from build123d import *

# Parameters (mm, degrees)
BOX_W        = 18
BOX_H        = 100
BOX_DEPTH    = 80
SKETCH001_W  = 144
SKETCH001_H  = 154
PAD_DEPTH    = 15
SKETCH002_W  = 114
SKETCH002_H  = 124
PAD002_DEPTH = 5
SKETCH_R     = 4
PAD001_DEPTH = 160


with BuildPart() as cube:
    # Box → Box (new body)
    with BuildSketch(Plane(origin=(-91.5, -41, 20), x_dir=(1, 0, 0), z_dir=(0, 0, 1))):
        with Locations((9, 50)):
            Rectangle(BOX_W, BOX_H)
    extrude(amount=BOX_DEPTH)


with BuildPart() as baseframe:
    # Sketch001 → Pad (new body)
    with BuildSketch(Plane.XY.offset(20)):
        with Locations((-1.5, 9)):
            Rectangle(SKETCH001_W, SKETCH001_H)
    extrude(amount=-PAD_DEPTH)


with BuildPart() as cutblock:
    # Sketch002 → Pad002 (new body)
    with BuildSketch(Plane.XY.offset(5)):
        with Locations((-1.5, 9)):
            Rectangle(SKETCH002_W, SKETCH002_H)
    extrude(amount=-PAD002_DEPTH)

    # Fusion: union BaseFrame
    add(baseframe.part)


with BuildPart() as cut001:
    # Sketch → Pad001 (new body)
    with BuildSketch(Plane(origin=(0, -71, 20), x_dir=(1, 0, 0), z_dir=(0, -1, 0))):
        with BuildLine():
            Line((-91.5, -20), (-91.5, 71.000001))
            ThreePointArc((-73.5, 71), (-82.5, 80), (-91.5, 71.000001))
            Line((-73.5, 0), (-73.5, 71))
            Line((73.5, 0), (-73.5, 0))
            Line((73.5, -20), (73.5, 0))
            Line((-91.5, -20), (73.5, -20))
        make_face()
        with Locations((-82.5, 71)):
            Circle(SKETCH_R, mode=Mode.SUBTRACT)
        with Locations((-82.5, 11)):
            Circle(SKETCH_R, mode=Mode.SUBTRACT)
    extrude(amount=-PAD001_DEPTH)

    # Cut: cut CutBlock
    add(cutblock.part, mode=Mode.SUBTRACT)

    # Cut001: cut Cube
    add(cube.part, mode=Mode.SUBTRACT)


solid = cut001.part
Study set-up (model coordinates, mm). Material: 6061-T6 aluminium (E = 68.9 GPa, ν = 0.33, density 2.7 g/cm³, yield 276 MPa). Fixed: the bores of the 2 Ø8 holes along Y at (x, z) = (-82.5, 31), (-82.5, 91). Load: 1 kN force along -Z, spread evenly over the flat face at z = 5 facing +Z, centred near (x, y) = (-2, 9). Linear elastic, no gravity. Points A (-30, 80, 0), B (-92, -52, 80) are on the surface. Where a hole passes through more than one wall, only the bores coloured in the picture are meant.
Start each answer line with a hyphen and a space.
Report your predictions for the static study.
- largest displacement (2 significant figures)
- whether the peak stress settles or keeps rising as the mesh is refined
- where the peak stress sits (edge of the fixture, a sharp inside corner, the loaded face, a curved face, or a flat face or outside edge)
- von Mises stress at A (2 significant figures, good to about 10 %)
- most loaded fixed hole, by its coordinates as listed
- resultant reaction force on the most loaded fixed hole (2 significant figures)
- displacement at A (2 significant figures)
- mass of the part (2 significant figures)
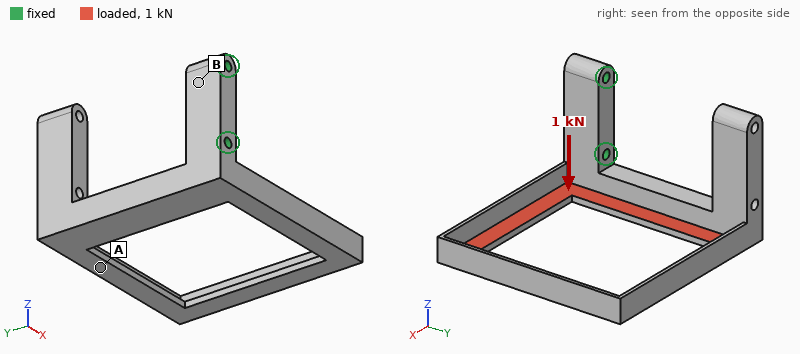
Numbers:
- 2.9 mm
- keeps rising
- a sharp inside corner
- 25 MPa
- (-82.5, 31)
- 1.0 kN
- 1.1 mm
- 550 g
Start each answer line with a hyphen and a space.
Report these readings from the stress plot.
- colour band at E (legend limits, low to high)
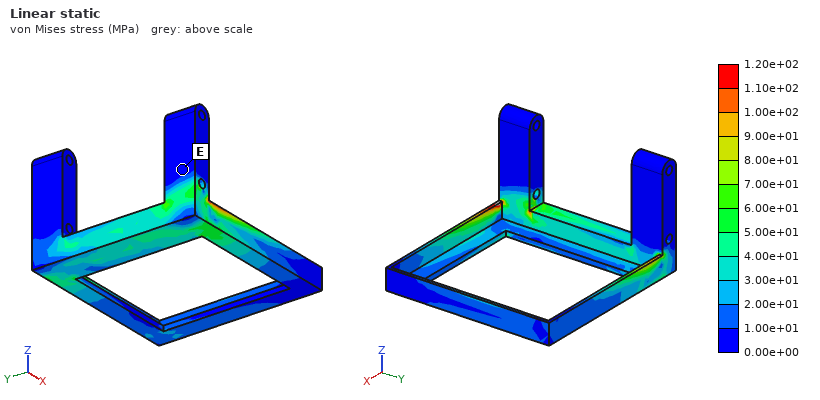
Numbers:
- 0.00e+00 to 1.00e+01 MPa
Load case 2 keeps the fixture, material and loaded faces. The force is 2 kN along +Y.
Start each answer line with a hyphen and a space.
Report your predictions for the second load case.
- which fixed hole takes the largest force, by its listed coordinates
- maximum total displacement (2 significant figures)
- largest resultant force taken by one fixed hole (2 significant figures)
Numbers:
- (-82.5, 31)
- 2.0 mm
- 2.0 kN
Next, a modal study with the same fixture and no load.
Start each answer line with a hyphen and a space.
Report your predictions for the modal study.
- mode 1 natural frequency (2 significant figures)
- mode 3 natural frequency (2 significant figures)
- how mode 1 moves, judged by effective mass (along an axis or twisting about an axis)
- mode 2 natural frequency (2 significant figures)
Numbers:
- 240 Hz
- 430 Hz
- along Z
- 300 Hz
